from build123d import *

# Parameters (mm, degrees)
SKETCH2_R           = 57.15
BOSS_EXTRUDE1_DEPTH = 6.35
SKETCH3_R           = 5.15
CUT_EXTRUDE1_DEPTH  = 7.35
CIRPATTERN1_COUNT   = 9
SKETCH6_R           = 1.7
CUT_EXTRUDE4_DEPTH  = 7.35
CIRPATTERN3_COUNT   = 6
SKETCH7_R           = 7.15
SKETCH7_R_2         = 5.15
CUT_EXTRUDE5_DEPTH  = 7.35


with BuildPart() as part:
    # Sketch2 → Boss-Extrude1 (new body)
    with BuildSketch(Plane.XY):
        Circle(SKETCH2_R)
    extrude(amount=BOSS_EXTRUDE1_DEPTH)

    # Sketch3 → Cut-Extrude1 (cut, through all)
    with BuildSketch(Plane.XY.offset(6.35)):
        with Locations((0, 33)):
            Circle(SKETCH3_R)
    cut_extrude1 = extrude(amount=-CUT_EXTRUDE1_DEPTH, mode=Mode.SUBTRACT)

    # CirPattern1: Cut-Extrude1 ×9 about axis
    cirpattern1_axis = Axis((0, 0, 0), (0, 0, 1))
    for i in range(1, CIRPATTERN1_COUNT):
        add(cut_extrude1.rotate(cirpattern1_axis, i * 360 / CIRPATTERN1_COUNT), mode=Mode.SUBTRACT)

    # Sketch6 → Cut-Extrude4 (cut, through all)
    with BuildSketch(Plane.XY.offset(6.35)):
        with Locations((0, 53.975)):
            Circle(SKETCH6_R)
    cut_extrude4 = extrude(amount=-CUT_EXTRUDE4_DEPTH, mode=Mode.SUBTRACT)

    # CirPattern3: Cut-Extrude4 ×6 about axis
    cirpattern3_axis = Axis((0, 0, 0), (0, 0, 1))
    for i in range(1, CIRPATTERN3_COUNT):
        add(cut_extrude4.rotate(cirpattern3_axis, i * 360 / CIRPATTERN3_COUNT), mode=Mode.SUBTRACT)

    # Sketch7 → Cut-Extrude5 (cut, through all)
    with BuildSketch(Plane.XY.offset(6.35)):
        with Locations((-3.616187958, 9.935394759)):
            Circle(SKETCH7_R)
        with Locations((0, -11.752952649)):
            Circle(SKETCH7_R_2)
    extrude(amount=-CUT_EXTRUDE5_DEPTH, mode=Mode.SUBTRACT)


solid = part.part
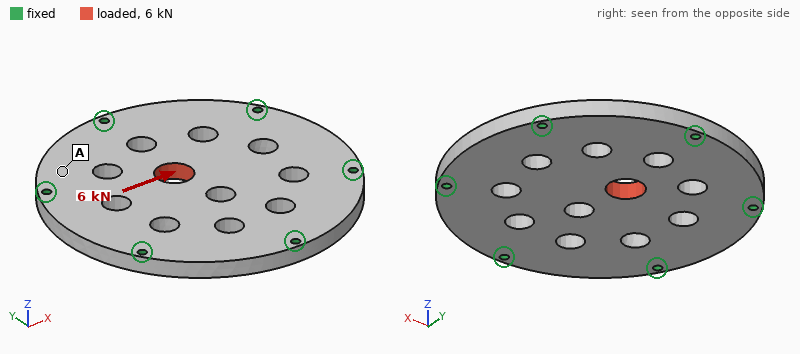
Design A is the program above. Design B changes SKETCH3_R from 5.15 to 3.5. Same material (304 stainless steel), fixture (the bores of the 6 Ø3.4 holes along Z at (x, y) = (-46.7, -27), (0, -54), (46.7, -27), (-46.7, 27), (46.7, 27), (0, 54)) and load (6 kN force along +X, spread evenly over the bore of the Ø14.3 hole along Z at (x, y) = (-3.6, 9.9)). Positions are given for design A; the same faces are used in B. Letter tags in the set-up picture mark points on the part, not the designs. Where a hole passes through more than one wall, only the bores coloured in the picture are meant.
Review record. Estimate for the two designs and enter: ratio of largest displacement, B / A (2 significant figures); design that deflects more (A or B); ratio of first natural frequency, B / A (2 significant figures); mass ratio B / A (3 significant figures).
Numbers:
0.89
A
1.0
1.04
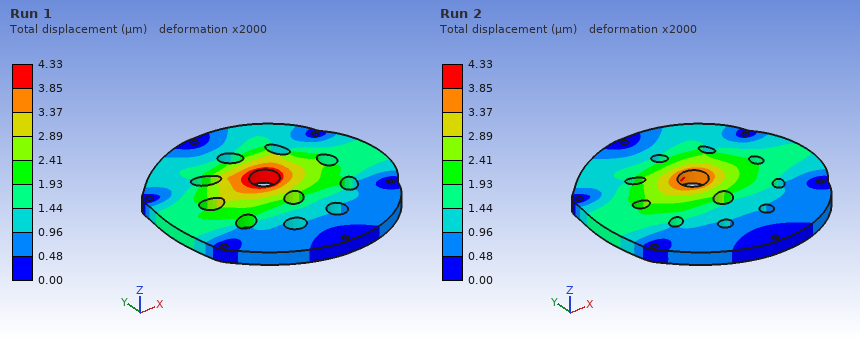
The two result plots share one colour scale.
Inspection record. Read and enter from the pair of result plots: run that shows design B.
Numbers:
Run 2
